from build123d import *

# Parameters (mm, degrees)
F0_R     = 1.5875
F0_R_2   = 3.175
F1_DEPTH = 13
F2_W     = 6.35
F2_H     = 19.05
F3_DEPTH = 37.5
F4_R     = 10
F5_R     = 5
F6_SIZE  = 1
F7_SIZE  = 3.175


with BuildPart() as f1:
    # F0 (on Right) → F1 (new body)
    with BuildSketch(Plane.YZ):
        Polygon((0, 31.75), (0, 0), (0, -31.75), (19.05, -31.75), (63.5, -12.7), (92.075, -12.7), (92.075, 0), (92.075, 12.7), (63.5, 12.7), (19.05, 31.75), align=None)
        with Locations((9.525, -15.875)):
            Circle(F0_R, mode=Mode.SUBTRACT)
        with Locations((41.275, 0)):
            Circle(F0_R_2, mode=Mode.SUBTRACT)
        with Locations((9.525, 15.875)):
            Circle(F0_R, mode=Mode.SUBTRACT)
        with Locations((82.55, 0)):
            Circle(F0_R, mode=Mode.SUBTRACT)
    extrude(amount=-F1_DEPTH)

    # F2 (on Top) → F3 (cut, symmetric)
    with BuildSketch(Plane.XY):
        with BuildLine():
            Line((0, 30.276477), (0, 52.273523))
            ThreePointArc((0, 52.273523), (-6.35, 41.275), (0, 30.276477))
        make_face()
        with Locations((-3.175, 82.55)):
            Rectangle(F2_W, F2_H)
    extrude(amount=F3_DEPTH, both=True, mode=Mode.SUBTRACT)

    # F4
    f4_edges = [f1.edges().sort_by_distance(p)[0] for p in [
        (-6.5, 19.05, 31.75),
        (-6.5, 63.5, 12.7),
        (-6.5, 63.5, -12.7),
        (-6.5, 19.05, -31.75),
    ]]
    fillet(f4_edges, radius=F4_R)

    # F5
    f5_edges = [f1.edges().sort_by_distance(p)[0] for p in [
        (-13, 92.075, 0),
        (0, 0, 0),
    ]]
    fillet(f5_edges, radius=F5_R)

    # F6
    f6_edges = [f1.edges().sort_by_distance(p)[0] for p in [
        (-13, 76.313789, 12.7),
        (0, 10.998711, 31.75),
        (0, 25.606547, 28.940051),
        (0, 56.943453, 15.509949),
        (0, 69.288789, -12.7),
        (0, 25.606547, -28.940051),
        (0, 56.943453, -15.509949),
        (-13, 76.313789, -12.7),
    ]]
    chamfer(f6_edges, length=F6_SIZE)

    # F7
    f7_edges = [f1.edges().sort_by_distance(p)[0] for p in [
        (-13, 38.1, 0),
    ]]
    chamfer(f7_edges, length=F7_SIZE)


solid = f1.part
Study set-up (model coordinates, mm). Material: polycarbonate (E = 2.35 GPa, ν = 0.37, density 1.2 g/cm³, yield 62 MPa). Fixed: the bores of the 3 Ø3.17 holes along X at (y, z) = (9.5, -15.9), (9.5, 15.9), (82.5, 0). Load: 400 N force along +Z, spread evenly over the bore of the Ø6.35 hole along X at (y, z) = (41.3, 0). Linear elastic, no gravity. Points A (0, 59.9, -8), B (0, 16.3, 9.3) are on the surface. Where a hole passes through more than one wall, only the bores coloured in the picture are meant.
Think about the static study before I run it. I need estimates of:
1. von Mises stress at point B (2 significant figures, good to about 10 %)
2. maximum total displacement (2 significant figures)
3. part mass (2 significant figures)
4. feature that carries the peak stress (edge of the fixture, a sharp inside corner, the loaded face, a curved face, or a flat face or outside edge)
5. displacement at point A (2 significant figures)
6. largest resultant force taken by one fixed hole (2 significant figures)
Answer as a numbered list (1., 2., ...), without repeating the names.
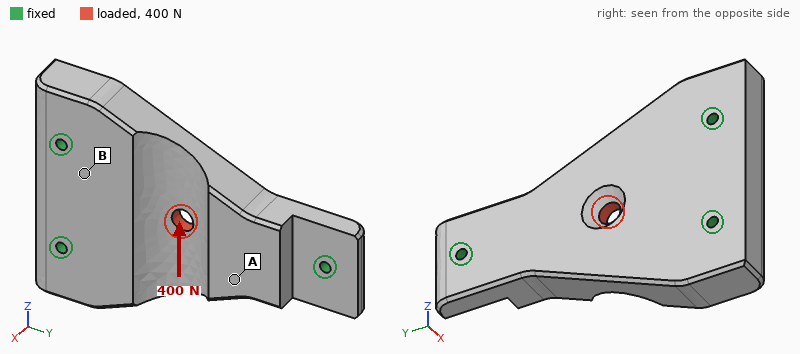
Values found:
1. 1.2 MPa
2. 53 µm
3. 51 g
4. the loaded face
5. 40 µm
6. 260 N
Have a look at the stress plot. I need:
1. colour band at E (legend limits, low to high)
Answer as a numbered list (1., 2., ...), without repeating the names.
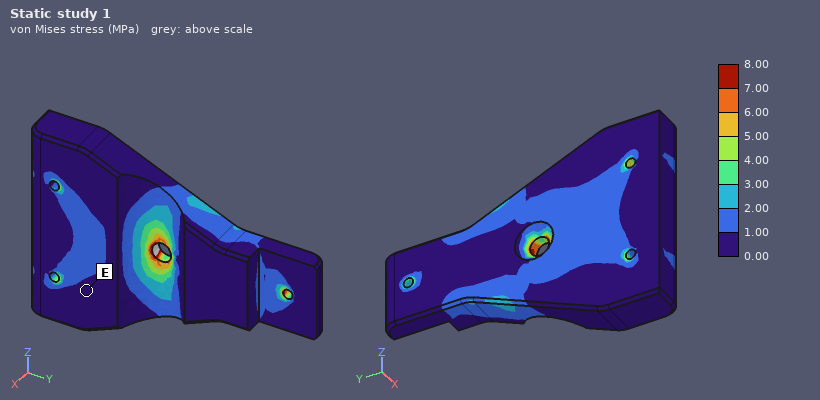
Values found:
1. 0.00 to 1.00 MPa
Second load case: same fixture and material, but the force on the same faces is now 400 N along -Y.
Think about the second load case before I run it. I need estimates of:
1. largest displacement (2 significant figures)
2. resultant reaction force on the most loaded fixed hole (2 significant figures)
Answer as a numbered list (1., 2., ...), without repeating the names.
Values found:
1. 25 µm
2. 150 N
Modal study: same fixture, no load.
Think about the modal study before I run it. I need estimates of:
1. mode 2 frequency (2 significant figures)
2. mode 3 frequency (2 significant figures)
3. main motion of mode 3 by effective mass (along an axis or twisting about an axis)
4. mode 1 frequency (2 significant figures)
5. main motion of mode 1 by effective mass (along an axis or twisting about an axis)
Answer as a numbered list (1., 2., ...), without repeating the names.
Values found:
1. 2800 Hz
2. 3600 Hz
3. along Z
4. 2000 Hz
5. along X
